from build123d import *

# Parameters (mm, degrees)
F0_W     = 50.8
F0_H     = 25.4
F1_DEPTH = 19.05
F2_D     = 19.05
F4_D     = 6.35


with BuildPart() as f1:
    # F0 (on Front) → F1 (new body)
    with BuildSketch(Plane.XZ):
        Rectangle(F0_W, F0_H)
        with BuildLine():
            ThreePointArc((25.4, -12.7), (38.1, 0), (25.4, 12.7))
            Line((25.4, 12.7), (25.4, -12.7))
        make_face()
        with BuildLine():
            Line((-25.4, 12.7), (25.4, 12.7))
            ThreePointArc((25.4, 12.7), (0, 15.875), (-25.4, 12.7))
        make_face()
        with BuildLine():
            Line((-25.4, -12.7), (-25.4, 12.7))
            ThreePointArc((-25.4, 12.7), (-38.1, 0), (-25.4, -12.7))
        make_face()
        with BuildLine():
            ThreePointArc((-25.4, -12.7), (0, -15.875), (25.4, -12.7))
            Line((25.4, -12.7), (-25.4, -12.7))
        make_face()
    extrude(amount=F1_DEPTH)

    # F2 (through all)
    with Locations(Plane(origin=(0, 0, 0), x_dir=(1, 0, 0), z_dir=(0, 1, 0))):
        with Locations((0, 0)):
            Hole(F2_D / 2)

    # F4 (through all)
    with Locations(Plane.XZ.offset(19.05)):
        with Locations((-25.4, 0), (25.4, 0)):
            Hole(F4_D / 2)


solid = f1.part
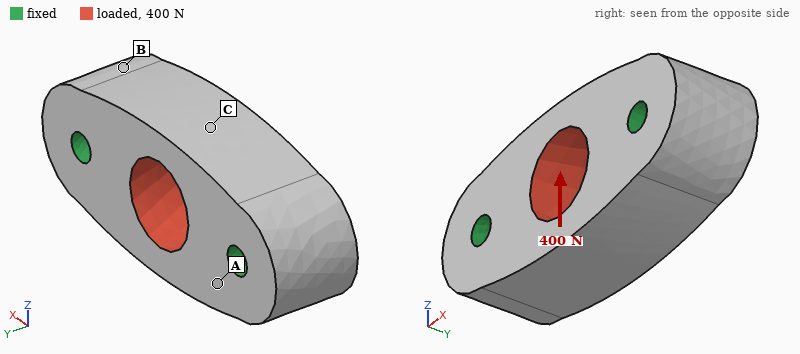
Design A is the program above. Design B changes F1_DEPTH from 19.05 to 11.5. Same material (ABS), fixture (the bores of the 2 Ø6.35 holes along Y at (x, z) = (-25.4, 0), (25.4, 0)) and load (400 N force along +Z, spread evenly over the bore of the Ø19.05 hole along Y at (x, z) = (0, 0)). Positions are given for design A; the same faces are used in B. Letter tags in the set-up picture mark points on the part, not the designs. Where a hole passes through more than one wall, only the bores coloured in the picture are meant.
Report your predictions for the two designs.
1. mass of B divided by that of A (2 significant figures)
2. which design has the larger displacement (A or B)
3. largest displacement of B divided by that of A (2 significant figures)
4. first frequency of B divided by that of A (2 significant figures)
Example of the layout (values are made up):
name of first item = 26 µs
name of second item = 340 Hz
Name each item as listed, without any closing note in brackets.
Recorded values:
mass of B divided by that of A = 0.60
which design has the larger displacement = B
largest displacement of B divided by that of A = 1.6
first frequency of B divided by that of A = 0.79
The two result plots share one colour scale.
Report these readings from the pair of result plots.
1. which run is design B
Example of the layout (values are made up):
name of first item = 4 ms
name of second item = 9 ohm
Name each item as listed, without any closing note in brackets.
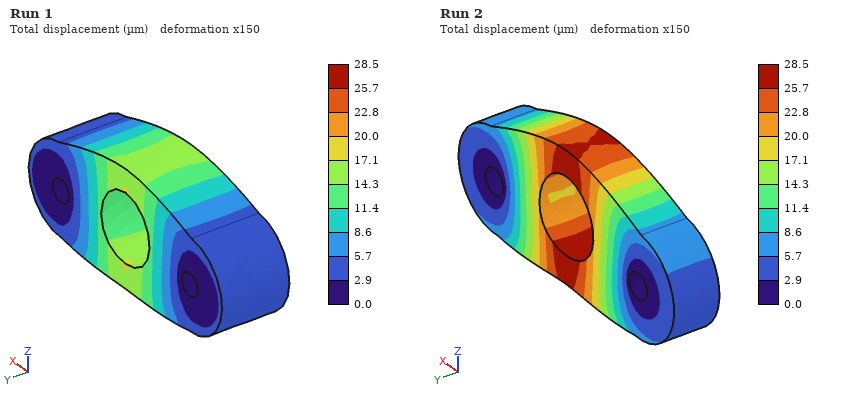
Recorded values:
which run is design B = Run 2
